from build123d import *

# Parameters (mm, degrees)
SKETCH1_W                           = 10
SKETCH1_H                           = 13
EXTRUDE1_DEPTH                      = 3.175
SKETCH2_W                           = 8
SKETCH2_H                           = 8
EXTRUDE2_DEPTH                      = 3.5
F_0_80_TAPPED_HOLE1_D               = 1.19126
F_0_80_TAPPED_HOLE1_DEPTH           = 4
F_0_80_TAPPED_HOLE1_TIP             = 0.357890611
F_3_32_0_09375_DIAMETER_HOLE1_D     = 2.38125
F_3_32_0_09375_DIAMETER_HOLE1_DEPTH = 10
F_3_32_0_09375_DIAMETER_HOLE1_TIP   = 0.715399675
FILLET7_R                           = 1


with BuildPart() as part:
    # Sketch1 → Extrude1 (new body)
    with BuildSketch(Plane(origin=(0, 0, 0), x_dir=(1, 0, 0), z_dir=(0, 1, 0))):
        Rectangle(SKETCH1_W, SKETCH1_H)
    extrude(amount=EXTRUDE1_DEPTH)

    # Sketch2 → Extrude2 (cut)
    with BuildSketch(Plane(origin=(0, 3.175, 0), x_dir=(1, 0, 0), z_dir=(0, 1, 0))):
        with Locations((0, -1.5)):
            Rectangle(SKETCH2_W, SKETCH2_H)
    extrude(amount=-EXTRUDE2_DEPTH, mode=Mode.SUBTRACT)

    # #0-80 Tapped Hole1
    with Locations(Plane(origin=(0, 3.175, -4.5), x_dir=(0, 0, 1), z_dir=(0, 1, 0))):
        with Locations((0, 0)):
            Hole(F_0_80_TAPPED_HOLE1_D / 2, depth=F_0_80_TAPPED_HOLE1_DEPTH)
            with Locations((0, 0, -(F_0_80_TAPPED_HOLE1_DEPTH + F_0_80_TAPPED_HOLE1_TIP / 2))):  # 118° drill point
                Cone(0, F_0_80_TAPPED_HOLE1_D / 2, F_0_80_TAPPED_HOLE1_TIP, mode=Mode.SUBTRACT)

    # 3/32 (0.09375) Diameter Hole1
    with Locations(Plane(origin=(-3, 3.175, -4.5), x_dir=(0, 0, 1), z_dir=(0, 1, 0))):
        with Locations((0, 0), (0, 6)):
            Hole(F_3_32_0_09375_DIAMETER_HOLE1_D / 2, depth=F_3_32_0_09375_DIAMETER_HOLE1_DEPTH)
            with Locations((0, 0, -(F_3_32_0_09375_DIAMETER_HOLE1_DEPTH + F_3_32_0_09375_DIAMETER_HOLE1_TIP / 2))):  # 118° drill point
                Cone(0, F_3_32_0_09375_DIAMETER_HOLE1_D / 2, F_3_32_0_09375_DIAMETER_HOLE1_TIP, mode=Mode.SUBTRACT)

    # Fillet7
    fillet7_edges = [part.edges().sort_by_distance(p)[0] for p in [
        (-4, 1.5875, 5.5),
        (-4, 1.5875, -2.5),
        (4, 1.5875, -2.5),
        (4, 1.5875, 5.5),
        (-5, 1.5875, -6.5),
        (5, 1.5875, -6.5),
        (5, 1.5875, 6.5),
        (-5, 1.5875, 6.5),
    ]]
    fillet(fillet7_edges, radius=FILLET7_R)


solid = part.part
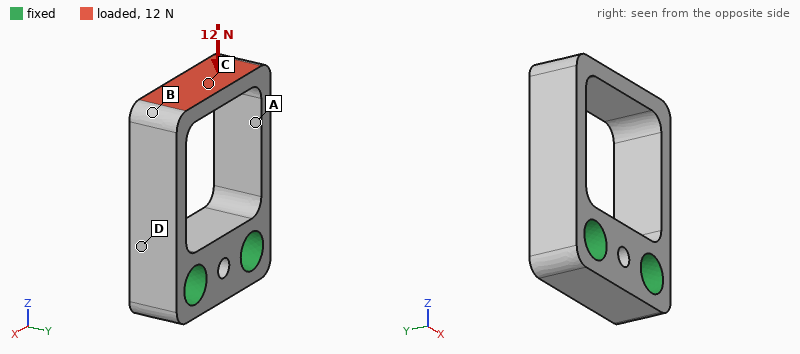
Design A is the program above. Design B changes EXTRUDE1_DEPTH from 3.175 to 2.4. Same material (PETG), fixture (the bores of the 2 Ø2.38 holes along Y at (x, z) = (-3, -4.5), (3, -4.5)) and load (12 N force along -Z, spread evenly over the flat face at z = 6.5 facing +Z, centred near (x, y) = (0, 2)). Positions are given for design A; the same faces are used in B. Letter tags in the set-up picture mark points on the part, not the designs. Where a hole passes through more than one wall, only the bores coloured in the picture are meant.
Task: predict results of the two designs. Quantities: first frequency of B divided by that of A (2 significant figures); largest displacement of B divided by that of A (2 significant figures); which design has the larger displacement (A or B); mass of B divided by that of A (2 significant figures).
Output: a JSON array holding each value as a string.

["0.99", "1.3", "B", "0.76"]
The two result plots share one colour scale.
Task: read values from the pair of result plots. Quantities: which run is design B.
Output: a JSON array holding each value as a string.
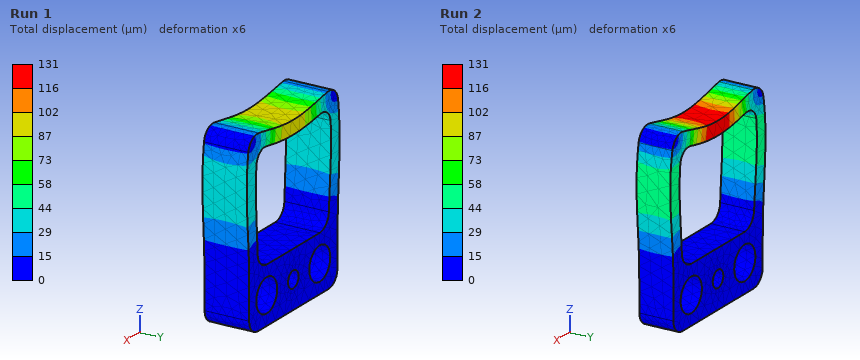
["Run 2"]
